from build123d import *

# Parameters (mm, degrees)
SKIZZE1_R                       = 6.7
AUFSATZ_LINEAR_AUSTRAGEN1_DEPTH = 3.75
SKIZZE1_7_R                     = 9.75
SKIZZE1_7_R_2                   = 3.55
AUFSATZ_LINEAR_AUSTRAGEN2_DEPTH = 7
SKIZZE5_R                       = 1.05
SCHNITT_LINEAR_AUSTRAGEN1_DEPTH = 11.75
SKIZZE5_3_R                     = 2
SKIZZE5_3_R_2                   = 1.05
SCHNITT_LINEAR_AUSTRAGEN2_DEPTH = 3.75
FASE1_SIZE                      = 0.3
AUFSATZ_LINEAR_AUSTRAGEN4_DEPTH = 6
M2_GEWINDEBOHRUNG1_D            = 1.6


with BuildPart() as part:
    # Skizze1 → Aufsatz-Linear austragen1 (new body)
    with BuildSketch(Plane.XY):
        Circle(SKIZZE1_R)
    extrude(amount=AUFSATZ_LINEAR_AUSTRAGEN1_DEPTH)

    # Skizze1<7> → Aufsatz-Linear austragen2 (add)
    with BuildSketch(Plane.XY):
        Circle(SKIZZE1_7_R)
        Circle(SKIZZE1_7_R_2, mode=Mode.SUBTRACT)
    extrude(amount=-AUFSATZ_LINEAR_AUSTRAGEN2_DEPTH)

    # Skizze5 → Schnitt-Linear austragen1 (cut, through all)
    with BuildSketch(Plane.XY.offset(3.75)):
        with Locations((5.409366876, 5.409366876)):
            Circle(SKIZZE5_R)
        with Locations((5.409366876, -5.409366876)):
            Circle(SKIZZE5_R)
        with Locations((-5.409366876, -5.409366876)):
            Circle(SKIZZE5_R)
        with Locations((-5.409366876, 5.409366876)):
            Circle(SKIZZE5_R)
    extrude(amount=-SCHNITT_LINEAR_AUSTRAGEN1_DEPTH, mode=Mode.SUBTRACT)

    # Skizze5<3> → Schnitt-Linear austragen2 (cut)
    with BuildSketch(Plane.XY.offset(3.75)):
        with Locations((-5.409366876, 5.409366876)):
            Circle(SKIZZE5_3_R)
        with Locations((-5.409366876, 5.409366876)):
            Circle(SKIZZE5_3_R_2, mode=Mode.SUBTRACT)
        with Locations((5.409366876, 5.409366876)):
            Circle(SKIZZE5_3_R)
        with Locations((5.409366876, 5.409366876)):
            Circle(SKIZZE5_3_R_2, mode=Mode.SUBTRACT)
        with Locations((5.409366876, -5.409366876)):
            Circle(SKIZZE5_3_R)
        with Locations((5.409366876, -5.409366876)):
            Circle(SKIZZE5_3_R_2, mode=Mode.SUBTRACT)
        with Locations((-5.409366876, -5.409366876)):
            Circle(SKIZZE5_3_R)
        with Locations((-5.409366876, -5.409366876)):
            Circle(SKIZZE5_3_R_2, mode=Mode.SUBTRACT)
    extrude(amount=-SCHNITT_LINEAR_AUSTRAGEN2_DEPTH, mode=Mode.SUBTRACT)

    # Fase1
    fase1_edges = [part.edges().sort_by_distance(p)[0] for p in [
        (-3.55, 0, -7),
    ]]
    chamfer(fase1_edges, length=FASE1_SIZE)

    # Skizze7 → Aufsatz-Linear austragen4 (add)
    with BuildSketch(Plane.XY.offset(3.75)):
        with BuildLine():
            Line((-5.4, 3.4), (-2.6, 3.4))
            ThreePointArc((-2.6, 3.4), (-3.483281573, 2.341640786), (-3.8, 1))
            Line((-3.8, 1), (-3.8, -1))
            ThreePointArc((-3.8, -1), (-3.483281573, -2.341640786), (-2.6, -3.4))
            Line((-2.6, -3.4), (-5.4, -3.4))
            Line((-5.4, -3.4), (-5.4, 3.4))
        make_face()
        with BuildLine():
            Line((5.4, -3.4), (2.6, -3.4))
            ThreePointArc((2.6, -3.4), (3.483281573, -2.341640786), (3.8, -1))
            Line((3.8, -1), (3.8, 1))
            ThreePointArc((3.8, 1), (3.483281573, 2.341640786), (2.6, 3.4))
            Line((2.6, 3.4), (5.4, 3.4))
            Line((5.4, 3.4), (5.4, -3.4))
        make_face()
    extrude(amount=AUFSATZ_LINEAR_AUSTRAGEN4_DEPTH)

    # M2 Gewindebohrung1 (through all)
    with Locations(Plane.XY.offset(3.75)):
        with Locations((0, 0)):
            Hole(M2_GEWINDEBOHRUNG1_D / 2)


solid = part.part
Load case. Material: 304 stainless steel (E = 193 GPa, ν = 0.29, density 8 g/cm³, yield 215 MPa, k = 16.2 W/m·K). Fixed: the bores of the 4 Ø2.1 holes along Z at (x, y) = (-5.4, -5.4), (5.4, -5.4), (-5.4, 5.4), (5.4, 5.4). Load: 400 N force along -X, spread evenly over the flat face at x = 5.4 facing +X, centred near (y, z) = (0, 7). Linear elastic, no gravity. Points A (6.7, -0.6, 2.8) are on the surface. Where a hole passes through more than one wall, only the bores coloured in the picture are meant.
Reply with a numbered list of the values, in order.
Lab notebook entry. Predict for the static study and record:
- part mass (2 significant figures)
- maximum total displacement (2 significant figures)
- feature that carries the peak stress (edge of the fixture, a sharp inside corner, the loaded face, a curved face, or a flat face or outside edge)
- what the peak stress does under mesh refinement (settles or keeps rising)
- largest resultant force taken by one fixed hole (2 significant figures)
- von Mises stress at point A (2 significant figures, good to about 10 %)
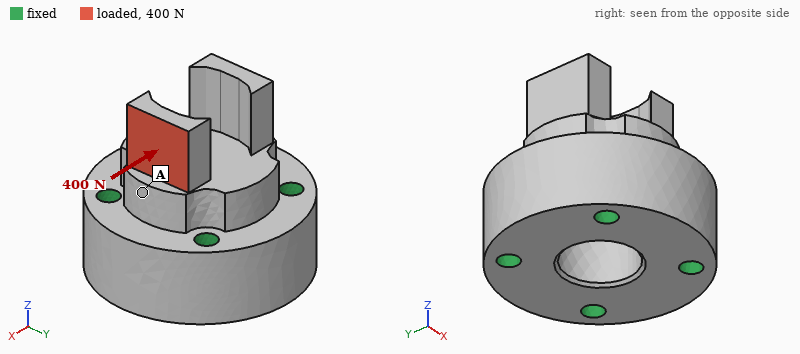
1. 19 g
2. 23 µm
3. a sharp inside corner
4. keeps rising
5. 200 N
6. 26 MPa
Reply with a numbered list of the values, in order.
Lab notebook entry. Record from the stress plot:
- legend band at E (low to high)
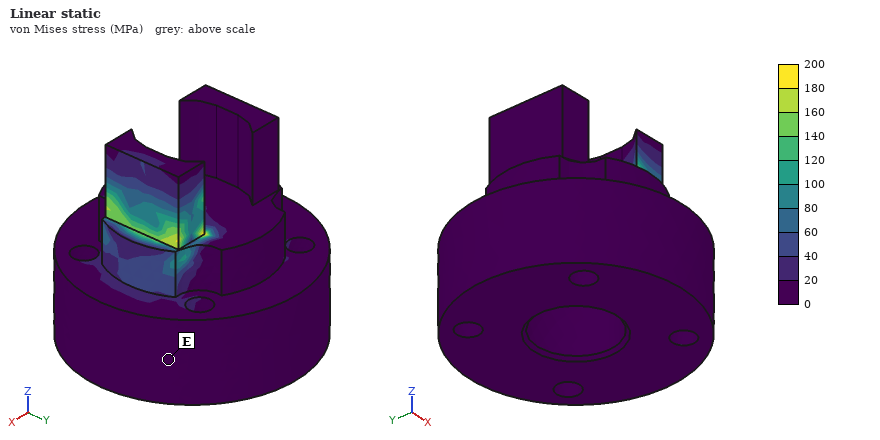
1. 0 to 20 MPa
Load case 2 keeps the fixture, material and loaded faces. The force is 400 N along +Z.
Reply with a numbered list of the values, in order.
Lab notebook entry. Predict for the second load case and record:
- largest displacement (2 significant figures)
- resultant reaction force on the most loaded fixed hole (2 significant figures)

1. 8.6 µm
2. 200 N
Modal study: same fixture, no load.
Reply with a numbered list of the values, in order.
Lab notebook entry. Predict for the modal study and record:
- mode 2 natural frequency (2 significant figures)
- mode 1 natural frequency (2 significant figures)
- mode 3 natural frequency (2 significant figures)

1. 34 kHz
2. 33 kHz
3. 53 kHz
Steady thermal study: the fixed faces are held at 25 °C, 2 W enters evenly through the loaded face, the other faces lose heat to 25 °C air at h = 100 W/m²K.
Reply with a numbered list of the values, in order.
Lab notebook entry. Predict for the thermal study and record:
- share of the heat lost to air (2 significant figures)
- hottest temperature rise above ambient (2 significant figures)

1. 25 %
2. 42 K
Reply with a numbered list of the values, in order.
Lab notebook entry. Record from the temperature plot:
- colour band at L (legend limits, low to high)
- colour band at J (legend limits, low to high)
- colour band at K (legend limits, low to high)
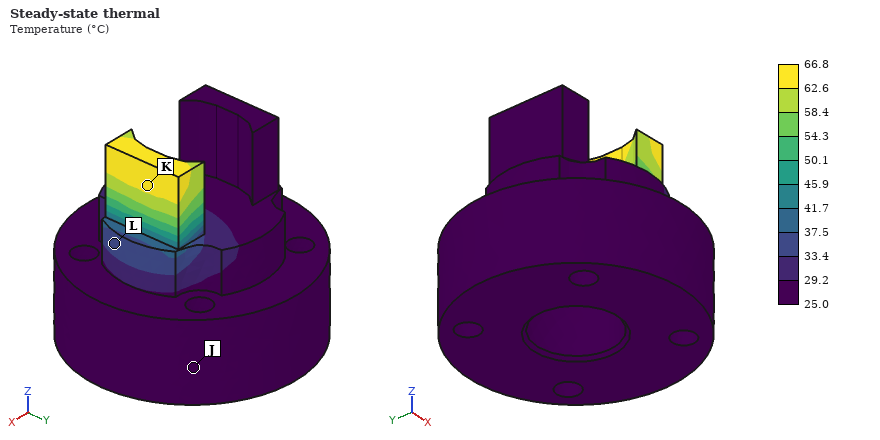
1. 33.4 to 37.5 °C
2. 25.0 to 29.2 °C
3. 62.6 to 66.8 °C
